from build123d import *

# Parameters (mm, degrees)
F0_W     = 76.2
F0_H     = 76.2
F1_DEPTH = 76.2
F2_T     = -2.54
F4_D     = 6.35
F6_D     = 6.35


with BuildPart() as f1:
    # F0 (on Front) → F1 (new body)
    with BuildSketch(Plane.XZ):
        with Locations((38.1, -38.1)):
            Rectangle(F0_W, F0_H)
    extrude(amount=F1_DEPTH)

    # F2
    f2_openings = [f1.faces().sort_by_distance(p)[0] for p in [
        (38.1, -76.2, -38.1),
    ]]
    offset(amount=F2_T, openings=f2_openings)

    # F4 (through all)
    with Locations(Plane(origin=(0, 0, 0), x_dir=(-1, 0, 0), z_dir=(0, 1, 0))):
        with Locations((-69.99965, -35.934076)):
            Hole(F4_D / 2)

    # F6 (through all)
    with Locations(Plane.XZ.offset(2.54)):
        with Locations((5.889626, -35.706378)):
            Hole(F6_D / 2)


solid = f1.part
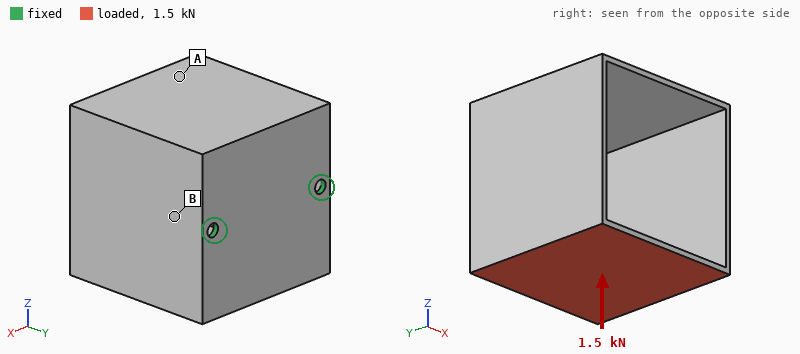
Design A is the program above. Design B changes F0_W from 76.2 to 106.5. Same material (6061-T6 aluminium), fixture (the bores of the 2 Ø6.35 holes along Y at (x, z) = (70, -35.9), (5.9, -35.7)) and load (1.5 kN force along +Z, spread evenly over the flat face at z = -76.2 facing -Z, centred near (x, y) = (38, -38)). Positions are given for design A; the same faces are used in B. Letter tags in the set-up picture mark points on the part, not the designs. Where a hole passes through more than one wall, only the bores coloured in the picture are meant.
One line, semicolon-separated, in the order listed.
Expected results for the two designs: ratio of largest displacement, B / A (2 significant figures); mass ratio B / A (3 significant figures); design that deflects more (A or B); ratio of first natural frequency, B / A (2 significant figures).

2.5; 1.25; B; 0.56
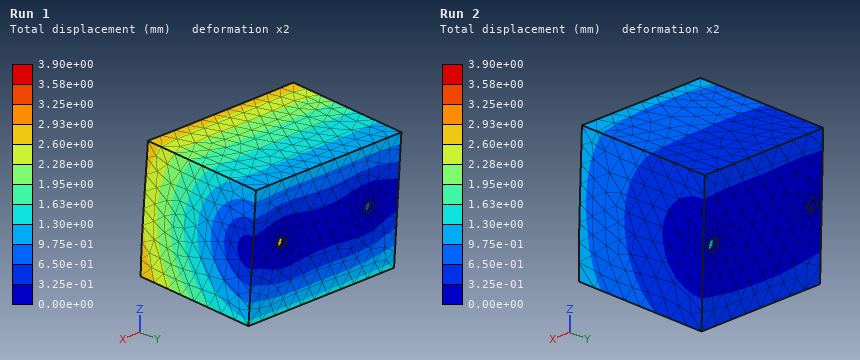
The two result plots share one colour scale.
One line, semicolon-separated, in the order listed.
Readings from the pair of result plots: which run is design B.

Run 1
